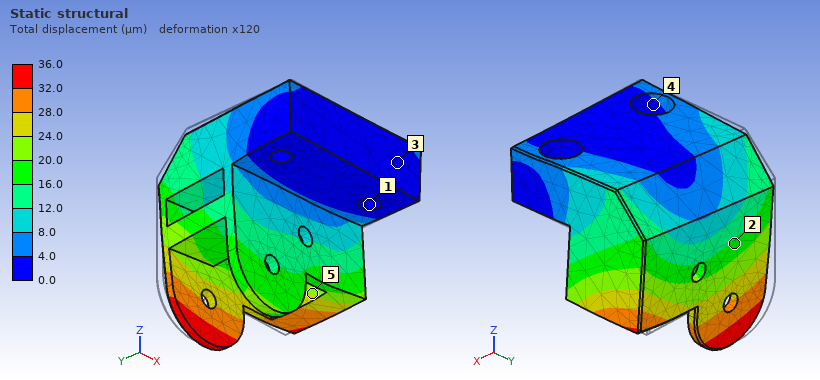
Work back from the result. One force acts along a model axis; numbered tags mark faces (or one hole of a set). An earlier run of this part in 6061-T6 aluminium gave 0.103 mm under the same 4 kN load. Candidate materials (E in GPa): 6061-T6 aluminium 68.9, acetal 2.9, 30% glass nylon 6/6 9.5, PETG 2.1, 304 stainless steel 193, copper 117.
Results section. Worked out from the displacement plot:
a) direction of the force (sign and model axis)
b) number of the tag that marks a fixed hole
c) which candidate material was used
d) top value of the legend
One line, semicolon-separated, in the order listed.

+X; 1; 304 stainless steel; 36.0 µm
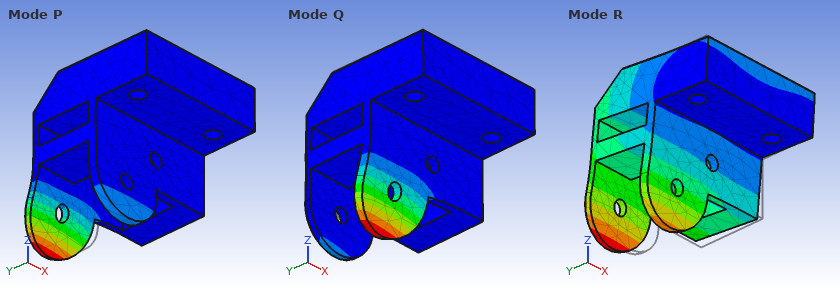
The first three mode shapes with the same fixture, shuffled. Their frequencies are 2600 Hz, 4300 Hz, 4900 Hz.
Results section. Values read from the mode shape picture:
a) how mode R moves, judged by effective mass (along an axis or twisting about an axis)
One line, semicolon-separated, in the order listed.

along Z
